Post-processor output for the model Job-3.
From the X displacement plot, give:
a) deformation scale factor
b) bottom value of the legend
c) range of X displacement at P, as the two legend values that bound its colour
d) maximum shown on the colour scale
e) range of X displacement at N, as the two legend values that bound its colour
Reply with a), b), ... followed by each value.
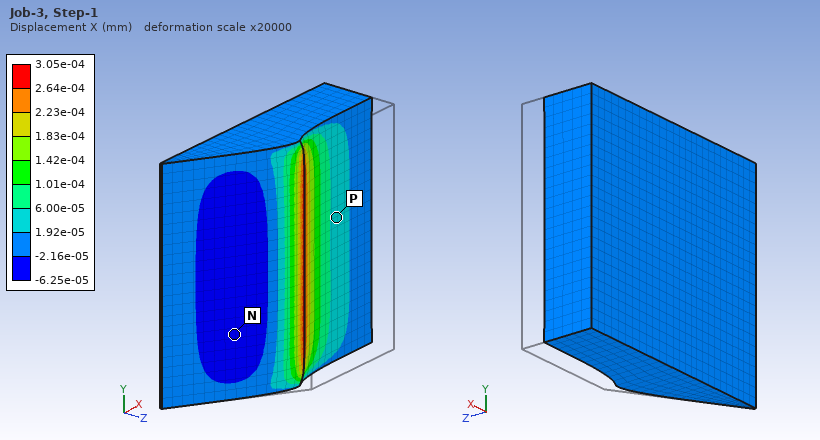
a) 20000
b) -6.25e-05 mm
c) 1.92e-05 to 6.00e-05 mm
d) 3.05e-04 mm
e) -6.25e-05 to -2.16e-05 mm
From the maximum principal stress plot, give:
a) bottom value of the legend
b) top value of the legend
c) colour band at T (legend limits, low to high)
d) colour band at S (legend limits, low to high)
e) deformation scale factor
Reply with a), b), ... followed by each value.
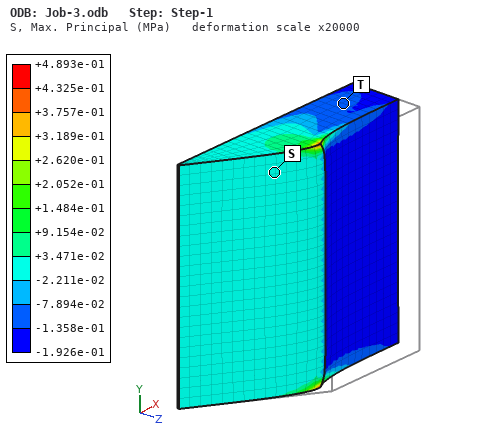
a) -1.926e-01 MPa
b) +4.893e-01 MPa
c) -1.358e-01 to -7.894e-02 MPa
d) -2.211e-02 to +3.471e-02 MPa
e) 20000
